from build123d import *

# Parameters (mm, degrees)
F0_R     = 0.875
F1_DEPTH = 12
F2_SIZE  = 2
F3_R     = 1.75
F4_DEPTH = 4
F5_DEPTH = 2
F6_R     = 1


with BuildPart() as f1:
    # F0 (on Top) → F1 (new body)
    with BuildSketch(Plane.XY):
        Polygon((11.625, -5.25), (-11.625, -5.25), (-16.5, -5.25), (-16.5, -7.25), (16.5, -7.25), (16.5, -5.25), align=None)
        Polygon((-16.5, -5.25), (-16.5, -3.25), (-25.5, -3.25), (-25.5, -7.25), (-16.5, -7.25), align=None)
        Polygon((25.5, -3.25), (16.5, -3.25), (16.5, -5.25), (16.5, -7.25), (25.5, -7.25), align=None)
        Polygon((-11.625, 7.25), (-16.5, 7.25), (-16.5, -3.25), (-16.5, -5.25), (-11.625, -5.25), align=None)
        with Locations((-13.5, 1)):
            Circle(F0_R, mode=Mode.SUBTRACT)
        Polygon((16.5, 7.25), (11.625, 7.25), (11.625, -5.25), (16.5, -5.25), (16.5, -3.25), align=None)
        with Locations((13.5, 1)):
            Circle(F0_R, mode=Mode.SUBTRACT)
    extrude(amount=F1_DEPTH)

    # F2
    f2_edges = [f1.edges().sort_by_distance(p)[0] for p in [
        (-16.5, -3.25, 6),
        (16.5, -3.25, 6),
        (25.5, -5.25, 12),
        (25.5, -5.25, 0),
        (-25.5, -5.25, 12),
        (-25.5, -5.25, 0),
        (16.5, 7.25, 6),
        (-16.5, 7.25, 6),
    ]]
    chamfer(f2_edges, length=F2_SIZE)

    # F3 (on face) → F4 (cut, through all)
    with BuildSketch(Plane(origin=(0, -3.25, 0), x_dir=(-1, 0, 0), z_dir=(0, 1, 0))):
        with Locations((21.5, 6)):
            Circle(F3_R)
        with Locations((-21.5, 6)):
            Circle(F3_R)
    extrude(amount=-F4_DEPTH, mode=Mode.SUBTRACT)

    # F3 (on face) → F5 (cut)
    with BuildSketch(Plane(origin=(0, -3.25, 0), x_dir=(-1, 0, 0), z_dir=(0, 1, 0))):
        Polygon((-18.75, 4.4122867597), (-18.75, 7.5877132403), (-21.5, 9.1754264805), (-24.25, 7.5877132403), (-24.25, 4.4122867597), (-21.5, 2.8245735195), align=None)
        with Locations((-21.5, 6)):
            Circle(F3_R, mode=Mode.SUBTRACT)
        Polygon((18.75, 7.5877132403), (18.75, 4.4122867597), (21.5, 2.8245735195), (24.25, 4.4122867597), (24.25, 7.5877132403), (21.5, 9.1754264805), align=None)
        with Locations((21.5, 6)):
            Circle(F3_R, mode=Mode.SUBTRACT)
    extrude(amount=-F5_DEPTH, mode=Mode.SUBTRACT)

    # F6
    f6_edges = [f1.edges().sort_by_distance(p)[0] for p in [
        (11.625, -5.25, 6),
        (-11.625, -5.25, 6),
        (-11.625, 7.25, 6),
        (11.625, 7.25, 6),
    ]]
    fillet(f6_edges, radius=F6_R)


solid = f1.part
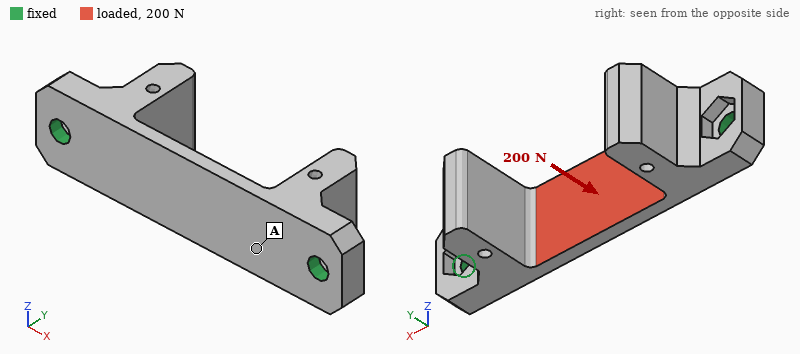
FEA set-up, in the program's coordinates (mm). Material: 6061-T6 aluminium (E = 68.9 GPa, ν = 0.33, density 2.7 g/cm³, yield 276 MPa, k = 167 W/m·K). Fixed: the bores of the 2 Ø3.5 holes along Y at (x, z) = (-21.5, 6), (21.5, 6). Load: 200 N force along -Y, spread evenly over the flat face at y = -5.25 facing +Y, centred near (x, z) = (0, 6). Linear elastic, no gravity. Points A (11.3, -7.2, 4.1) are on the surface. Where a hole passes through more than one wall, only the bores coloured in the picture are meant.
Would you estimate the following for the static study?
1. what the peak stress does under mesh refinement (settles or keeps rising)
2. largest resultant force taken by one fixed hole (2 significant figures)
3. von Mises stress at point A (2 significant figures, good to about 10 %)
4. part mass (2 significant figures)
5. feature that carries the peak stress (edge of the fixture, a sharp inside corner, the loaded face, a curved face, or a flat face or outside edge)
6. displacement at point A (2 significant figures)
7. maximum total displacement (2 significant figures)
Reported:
keeps rising
120 N
18 MPa
7.8 g
edge of the fixture
22 µm
51 µm
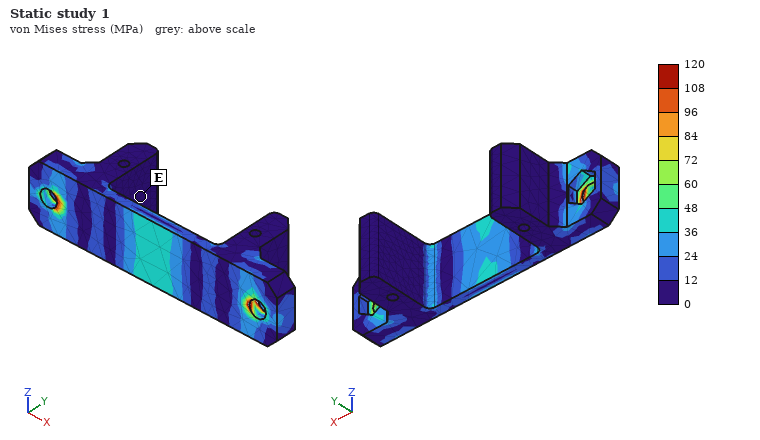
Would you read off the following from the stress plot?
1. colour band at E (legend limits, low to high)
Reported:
0 to 12 MPa
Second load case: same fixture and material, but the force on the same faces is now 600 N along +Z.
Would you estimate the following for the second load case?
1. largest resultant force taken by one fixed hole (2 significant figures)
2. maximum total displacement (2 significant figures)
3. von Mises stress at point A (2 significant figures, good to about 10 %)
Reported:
300 N
27 µm
17 MPa
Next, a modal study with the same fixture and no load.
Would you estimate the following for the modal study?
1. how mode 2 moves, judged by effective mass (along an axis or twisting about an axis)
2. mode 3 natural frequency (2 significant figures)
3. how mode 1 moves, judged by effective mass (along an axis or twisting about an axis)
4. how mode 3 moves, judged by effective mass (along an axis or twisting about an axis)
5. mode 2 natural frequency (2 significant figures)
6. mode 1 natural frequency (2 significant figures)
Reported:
along X
10000 Hz
along Y
along Z
9400 Hz
6300 Hz
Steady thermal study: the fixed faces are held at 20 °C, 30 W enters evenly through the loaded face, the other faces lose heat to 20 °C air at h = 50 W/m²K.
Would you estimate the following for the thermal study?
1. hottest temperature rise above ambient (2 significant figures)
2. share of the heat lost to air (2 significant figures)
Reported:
44 K
5.6 %
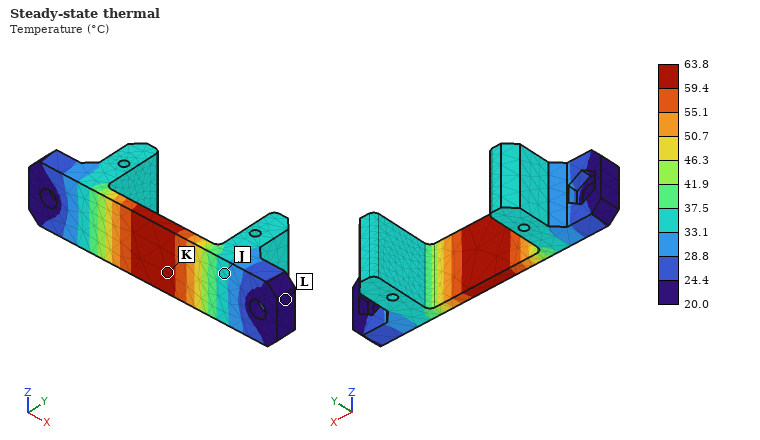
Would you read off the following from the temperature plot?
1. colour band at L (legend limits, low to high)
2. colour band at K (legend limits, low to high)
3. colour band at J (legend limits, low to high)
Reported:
20.0 to 24.4 °C
59.4 to 63.8 °C
33.1 to 37.5 °C
